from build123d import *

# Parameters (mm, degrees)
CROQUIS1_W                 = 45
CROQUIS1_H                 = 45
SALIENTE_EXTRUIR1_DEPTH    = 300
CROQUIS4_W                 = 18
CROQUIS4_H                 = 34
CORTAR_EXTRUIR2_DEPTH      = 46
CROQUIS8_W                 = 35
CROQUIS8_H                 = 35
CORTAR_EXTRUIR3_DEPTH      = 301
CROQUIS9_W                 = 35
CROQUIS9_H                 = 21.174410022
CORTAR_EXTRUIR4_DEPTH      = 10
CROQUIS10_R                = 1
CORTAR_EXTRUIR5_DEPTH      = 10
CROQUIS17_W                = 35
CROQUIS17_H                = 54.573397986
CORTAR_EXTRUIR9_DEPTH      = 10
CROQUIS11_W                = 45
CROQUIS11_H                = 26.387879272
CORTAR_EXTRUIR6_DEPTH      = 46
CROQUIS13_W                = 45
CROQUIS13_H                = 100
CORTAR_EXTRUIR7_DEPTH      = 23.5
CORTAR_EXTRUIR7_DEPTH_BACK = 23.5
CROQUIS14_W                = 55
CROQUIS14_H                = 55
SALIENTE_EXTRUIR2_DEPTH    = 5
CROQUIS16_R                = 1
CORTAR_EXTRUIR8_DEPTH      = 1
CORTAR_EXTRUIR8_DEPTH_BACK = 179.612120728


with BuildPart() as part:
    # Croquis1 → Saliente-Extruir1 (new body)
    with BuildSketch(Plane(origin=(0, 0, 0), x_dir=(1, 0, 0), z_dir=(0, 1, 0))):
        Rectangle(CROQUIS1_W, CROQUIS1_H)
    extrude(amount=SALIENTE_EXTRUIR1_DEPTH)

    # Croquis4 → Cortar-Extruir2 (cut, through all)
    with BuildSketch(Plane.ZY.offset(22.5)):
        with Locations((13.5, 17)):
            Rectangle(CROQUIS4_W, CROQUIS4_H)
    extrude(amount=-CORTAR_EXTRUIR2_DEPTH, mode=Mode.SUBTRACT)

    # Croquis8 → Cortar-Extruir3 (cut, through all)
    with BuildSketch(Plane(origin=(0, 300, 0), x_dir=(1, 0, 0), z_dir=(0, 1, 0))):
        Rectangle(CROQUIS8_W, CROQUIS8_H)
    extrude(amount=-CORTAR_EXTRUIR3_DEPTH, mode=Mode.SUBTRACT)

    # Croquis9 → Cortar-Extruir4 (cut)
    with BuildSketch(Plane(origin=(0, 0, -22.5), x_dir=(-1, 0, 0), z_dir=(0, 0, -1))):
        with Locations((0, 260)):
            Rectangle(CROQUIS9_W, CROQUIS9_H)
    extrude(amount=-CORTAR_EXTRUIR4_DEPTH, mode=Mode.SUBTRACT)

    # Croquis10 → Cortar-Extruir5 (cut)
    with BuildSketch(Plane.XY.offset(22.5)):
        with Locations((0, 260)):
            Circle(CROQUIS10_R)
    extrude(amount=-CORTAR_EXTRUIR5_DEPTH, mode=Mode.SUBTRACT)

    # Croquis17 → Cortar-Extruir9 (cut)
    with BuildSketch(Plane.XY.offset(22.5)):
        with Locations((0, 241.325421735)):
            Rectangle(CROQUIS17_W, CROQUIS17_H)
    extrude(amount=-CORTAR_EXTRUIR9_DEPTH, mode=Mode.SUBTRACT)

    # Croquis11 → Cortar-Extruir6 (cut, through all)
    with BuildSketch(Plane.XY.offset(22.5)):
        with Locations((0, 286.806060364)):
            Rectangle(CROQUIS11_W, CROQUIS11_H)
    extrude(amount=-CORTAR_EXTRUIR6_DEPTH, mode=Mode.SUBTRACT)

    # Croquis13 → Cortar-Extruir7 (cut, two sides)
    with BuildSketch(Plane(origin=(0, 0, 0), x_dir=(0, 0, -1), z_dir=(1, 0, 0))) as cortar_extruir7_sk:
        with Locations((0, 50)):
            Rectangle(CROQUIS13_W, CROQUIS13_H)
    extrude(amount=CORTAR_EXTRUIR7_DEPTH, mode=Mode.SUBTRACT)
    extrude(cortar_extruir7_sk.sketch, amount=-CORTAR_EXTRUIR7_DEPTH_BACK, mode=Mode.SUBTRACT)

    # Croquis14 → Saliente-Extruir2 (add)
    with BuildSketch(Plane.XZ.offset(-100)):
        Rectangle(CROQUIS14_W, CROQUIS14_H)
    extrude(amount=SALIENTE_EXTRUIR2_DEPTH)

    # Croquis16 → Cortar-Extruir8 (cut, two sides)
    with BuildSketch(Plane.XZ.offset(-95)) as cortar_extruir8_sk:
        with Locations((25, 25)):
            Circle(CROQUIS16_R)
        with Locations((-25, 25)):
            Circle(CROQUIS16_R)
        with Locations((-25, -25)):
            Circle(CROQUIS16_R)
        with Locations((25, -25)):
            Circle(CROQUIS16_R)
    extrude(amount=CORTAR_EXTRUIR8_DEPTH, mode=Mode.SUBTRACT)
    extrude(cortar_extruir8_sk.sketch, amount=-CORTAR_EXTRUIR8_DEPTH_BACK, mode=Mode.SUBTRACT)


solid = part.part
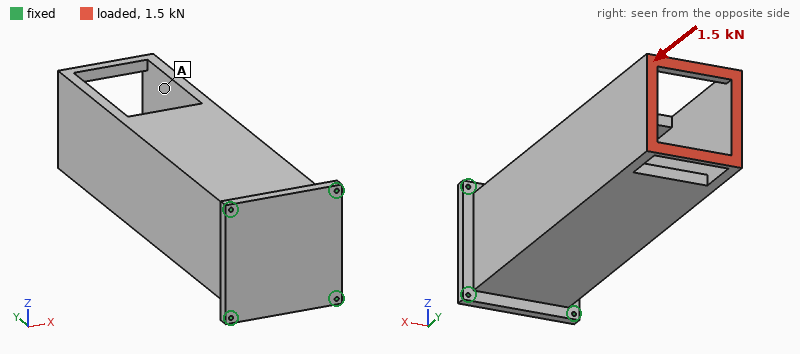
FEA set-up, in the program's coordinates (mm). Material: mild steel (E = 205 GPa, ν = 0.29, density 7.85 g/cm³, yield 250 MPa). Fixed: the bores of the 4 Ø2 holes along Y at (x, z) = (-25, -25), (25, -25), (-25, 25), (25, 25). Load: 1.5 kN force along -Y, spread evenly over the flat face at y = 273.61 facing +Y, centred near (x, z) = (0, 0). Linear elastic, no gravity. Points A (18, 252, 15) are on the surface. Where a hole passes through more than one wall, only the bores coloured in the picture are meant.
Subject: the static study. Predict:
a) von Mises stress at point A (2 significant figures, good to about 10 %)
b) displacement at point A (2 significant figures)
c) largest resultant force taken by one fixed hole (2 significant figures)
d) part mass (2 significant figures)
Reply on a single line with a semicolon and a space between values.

8.6 MPa; 4.8 µm; 400 N; 1.1 kg
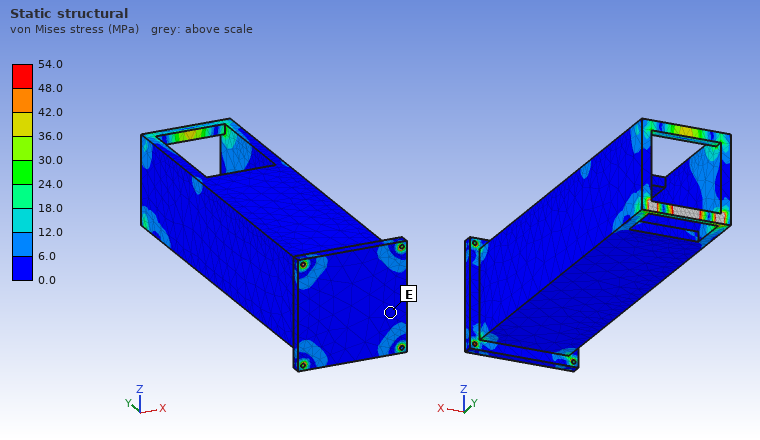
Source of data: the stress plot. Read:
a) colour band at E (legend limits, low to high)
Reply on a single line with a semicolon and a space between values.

0.0 to 6.0 MPa
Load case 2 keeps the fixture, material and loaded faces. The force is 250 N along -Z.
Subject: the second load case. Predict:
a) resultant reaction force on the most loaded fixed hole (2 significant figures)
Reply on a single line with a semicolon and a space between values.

490 N
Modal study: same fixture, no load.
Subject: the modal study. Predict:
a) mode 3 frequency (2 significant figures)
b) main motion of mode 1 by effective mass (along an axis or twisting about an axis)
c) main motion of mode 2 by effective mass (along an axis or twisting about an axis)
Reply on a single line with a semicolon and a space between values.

2400 Hz; along X; along Z
